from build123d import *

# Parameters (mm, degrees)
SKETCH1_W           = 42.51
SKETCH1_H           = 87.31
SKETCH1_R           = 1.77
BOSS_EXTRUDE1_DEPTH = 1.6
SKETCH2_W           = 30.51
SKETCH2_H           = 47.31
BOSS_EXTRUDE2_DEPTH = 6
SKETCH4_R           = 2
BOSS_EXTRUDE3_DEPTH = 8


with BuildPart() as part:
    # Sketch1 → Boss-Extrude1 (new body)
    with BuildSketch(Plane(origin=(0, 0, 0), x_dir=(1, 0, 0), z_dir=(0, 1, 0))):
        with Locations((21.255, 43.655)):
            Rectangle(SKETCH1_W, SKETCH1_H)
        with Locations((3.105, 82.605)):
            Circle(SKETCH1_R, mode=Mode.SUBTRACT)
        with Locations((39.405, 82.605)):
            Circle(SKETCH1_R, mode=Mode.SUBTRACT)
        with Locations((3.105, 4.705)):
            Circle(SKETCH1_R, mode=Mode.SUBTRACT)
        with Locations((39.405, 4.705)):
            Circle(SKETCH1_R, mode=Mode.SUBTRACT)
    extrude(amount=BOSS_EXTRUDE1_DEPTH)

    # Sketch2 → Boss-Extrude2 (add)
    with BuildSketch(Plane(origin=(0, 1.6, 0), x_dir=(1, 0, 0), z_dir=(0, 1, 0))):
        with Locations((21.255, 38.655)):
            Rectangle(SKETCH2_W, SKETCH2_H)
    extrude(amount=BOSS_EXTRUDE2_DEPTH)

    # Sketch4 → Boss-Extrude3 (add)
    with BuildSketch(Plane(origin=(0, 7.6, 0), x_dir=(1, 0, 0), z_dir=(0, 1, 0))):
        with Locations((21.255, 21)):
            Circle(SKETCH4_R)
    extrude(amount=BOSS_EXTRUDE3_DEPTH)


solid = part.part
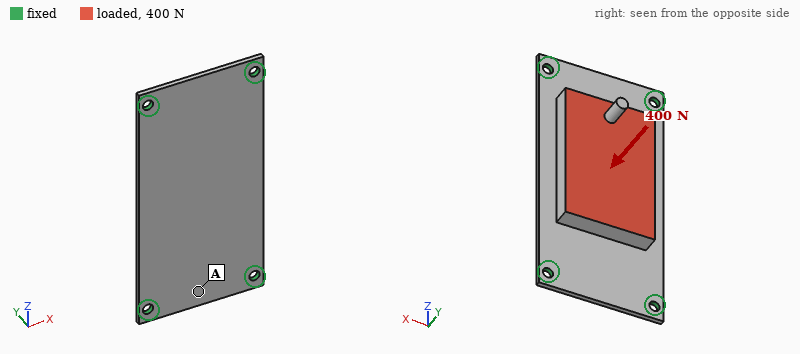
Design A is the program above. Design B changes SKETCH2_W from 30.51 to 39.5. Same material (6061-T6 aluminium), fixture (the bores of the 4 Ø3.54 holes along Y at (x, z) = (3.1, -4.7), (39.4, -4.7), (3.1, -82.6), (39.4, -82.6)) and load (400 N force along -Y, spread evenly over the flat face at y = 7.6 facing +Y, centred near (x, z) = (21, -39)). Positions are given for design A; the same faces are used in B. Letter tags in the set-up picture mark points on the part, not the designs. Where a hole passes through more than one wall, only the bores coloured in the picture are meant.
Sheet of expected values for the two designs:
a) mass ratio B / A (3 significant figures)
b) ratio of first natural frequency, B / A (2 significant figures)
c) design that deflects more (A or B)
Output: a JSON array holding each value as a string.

["1.17", "0.99", "A"]
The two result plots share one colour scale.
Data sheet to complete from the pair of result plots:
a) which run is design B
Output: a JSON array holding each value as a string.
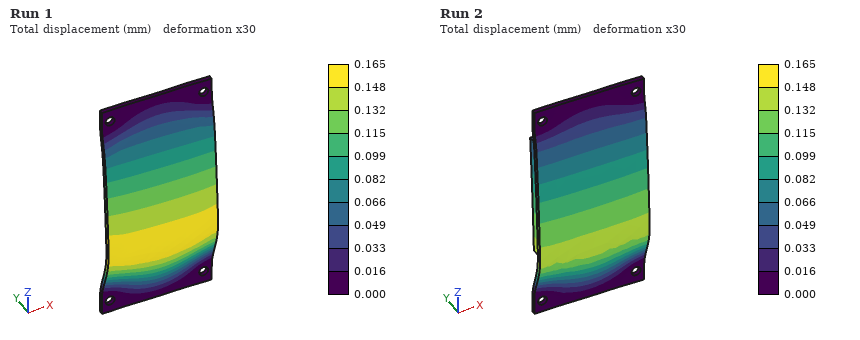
["Run 2"]
